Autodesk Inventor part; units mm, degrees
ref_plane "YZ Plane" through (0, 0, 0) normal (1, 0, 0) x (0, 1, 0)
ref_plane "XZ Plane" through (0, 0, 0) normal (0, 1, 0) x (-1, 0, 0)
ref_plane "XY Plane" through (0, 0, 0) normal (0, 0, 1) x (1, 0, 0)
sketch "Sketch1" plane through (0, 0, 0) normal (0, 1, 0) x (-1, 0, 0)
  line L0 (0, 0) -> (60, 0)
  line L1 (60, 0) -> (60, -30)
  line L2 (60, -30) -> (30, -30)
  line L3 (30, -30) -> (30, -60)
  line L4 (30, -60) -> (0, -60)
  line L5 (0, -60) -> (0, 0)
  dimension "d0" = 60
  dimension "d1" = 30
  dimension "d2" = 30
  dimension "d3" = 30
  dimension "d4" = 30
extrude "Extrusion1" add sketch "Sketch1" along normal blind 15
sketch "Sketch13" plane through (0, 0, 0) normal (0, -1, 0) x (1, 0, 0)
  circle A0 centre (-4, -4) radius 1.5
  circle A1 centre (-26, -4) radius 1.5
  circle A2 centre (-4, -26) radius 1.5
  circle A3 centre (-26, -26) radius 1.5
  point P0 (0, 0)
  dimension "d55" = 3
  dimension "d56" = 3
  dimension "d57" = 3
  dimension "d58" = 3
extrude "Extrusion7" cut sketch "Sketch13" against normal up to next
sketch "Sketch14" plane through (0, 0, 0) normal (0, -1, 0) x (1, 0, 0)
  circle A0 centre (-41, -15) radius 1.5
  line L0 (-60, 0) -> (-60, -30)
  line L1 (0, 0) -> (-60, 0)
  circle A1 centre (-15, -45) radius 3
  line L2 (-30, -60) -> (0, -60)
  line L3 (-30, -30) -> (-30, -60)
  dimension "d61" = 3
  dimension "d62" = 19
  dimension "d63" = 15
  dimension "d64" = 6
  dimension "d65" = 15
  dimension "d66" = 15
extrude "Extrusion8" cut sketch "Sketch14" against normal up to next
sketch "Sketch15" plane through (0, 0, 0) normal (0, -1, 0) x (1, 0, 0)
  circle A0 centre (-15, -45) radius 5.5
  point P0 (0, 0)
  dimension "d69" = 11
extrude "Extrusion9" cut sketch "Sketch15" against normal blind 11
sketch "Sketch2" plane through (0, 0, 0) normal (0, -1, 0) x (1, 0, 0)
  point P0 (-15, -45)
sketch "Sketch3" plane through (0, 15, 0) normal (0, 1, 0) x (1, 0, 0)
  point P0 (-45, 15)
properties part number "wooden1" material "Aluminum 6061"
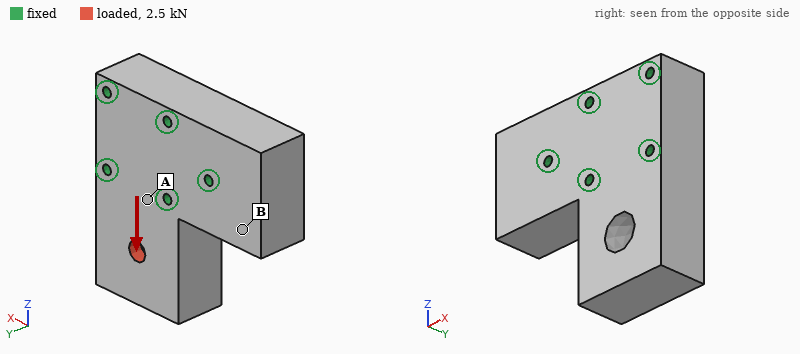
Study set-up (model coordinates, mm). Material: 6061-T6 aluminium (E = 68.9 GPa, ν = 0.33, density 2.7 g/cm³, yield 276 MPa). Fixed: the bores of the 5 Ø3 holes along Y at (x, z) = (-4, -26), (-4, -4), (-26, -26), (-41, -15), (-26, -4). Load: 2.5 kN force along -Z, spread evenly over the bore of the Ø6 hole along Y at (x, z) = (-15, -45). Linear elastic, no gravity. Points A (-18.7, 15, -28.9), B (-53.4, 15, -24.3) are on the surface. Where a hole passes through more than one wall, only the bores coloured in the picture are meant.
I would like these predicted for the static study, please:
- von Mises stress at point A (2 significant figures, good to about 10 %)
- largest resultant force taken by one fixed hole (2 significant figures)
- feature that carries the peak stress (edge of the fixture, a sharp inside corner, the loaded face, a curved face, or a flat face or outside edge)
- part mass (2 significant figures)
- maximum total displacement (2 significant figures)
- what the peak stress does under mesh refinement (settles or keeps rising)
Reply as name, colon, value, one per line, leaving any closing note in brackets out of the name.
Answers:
von Mises stress at point A: 12 MPa
largest resultant force taken by one fixed hole: 1.1 kN
feature that carries the peak stress: a sharp inside corner
part mass: 100 g
maximum total displacement: 14 µm
what the peak stress does under mesh refinement: keeps rising
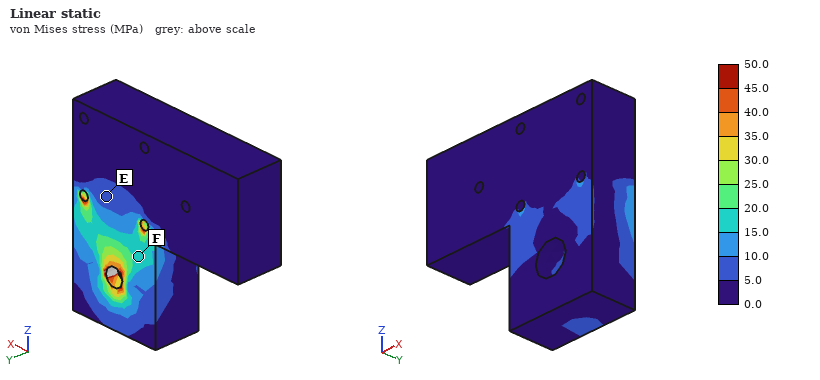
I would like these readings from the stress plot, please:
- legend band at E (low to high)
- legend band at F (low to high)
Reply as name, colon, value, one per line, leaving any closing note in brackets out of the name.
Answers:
legend band at E: 5.0 to 10.0 MPa
legend band at F: 15.0 to 20.0 MPa
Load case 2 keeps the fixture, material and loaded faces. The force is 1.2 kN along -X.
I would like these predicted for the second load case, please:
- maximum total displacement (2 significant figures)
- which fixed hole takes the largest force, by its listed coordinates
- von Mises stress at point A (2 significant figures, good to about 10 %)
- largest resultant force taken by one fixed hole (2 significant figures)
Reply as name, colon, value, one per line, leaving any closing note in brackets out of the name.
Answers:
maximum total displacement: 7.6 µm
which fixed hole takes the largest force, by its listed coordinates: (-4, -26)
von Mises stress at point A: 7.1 MPa
largest resultant force taken by one fixed hole: 1.1 kN
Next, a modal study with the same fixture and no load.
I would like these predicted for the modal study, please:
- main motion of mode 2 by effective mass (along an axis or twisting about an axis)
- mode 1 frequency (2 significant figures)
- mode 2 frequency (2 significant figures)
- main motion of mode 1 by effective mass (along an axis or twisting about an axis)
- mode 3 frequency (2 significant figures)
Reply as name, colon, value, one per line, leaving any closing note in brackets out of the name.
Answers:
main motion of mode 2 by effective mass: along X
mode 1 frequency: 8600 Hz
mode 2 frequency: 14 kHz
main motion of mode 1 by effective mass: along Y
mode 3 frequency: 17 kHz
